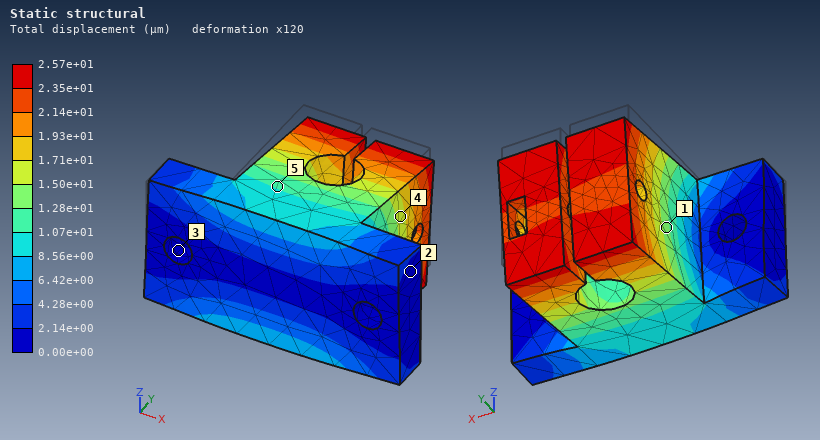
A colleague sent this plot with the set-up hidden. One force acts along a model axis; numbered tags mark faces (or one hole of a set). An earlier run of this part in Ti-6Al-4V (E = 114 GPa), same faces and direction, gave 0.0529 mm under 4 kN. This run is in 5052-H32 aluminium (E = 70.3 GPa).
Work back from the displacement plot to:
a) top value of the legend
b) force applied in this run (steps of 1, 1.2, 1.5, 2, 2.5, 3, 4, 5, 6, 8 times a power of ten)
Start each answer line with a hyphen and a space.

- 2.57e+01 µm
- 1.2 kN
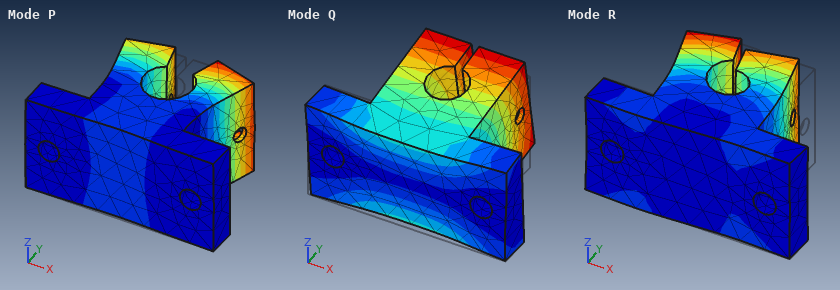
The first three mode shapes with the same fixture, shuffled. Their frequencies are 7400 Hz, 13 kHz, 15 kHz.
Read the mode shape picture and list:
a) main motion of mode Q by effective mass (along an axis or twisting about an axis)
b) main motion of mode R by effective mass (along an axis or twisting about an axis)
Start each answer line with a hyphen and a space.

- along Z
- along X
